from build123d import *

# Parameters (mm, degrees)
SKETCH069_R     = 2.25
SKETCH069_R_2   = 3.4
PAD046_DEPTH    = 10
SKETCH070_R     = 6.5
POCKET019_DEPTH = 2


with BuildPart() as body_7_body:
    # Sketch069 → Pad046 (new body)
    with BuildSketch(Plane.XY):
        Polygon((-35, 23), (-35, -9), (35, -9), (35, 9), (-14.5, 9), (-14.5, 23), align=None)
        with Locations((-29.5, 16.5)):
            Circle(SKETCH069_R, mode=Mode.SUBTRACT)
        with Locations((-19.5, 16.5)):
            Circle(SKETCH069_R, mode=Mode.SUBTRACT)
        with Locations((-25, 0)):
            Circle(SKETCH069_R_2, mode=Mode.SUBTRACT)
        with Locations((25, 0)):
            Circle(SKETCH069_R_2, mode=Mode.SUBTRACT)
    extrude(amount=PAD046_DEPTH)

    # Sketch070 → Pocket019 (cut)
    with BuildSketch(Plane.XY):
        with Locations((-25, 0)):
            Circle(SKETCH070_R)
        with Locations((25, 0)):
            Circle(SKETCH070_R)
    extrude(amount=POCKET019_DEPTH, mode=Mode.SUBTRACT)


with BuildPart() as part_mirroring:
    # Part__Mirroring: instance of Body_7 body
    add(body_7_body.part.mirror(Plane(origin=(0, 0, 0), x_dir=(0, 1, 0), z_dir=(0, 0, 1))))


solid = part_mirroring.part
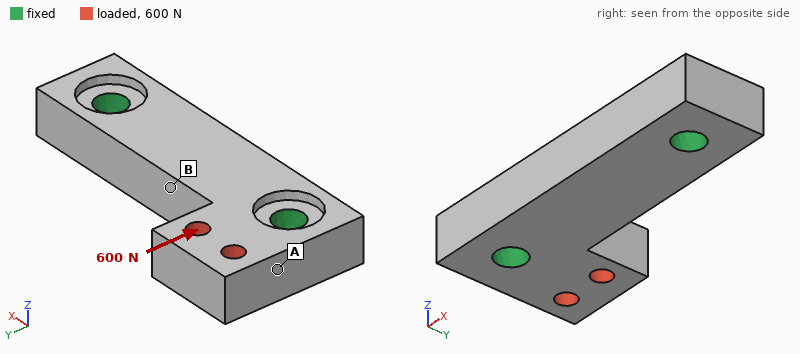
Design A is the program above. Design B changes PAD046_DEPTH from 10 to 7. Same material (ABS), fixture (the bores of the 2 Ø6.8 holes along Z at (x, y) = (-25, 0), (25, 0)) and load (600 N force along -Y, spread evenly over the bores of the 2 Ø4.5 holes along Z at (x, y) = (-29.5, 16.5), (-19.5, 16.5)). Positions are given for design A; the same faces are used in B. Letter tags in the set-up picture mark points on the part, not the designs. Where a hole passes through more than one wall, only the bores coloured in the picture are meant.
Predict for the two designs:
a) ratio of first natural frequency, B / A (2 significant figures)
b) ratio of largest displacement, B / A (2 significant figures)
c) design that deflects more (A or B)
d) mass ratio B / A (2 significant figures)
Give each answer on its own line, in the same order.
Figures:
0.73
2.1
B
0.69
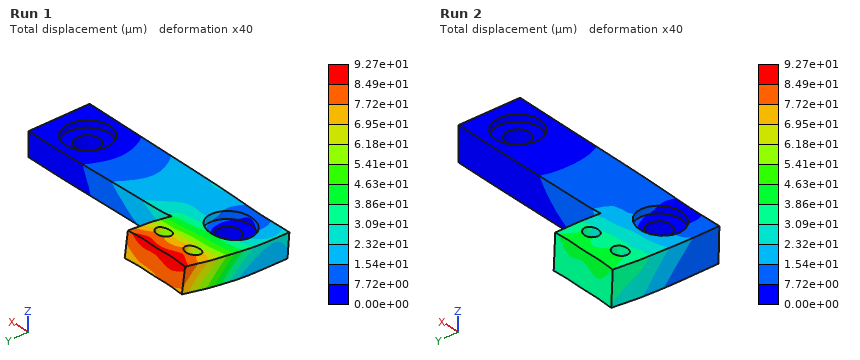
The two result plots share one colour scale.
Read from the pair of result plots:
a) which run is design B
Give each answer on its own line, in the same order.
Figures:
Run 1
